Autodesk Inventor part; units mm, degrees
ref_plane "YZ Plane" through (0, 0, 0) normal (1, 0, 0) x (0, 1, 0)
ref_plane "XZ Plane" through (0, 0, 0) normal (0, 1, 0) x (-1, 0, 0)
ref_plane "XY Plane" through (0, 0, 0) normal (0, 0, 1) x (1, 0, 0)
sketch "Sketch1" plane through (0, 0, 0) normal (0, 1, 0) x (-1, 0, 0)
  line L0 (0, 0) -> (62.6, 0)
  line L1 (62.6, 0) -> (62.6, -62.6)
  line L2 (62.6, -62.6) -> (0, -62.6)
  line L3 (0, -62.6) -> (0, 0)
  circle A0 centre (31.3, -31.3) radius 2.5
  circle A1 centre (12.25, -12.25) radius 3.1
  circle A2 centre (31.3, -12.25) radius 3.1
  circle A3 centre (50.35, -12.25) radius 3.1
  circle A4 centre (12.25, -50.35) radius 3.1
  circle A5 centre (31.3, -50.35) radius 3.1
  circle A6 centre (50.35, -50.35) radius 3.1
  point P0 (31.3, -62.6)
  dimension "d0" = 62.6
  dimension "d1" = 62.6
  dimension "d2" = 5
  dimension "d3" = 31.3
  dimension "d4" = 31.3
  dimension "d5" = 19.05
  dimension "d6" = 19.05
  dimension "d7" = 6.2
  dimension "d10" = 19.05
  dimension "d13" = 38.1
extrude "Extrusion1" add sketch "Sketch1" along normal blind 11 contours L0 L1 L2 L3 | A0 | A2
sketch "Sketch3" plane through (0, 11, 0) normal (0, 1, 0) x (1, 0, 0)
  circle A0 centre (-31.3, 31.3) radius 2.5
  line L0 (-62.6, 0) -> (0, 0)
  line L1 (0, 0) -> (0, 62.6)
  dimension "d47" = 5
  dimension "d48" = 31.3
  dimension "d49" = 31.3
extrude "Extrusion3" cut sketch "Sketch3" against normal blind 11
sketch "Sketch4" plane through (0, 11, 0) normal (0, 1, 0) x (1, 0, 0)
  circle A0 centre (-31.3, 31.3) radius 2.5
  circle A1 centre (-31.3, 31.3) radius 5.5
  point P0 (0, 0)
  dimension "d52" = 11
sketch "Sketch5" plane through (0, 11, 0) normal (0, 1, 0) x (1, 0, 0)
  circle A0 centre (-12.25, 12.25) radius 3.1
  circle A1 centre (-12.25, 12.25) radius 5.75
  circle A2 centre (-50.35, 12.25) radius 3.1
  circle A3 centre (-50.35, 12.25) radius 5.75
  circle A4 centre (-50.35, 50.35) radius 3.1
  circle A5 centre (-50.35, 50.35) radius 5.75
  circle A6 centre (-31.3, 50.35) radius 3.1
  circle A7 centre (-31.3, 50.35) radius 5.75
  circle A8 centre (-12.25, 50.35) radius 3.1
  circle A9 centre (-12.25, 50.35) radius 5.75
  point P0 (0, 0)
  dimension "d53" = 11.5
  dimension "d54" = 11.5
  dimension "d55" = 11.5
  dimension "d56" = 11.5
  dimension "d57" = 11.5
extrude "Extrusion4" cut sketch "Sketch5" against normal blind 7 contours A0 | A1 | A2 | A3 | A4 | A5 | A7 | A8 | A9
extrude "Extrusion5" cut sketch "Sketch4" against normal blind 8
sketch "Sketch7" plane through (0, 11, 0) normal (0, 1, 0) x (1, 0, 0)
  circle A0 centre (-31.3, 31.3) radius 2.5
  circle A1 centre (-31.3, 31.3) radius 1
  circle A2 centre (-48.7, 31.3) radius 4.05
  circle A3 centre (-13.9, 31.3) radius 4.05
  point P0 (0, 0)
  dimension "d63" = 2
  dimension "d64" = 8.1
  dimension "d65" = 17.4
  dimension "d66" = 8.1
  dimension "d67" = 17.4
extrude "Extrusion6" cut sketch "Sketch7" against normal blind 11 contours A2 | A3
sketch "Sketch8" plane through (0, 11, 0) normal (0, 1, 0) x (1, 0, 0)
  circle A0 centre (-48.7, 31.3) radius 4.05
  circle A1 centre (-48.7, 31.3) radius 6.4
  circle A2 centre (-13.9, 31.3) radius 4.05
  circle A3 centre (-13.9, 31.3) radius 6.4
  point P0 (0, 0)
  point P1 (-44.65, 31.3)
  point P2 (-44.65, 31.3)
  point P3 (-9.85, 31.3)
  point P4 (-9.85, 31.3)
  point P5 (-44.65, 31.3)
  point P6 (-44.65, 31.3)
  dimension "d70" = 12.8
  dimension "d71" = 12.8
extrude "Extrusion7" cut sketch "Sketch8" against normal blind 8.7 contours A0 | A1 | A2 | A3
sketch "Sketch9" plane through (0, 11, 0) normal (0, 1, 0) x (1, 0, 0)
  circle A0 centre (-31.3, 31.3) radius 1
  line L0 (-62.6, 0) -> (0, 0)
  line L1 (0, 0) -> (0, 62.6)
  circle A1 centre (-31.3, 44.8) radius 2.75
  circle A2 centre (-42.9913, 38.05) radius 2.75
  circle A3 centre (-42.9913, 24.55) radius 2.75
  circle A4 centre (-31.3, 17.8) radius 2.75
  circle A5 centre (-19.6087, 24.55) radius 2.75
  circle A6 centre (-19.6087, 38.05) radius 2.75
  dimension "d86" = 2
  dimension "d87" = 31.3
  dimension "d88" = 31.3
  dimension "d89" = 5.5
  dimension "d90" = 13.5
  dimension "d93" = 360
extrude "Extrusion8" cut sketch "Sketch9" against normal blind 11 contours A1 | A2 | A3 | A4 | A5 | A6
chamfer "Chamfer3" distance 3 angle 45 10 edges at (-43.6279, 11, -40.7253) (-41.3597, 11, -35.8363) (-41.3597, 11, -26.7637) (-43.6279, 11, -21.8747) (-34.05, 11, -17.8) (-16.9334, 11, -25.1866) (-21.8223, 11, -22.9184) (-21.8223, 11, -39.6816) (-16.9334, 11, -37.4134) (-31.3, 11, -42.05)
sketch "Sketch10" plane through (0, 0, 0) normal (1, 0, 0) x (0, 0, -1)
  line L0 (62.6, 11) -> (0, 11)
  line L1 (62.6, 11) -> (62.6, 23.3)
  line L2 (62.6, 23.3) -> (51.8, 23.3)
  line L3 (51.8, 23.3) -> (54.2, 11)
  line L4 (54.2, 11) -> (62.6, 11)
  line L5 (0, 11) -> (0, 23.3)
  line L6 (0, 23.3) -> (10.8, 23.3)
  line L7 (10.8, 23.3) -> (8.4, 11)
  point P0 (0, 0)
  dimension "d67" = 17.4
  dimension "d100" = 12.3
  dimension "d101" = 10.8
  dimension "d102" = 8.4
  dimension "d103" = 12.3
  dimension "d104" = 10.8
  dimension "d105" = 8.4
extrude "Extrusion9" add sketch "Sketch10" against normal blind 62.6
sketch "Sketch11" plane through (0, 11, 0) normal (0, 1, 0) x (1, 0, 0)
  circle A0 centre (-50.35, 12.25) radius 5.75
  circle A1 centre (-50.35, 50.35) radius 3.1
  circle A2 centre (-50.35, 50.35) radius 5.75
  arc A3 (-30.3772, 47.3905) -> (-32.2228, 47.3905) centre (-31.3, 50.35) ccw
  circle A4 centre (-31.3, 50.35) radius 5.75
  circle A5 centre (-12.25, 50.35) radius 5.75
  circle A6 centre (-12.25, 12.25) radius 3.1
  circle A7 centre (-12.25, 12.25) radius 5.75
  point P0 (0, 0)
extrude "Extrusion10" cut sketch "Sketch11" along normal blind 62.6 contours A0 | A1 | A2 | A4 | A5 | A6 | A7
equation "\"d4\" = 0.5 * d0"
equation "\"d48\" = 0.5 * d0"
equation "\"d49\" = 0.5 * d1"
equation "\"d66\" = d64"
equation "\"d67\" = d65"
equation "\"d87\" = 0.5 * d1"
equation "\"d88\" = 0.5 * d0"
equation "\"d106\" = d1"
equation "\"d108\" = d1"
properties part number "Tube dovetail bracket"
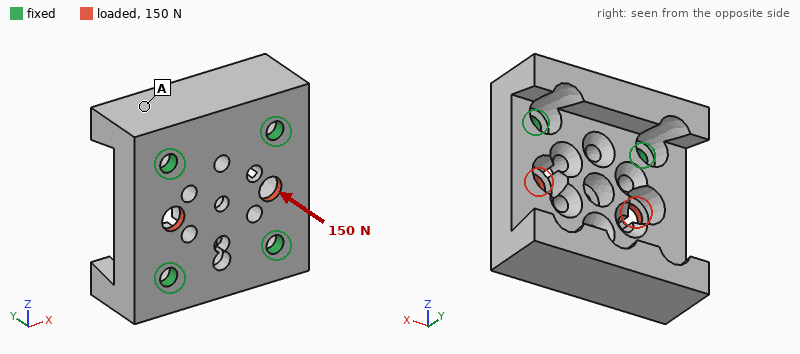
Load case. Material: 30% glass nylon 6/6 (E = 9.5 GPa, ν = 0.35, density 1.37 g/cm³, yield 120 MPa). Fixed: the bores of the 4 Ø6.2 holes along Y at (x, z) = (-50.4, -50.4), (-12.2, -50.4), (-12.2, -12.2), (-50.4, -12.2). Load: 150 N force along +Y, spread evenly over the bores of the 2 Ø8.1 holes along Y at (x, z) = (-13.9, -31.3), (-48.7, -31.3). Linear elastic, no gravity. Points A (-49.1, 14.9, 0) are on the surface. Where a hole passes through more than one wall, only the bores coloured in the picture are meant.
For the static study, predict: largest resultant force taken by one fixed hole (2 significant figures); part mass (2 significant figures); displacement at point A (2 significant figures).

44 N
64 g
2.4 µm
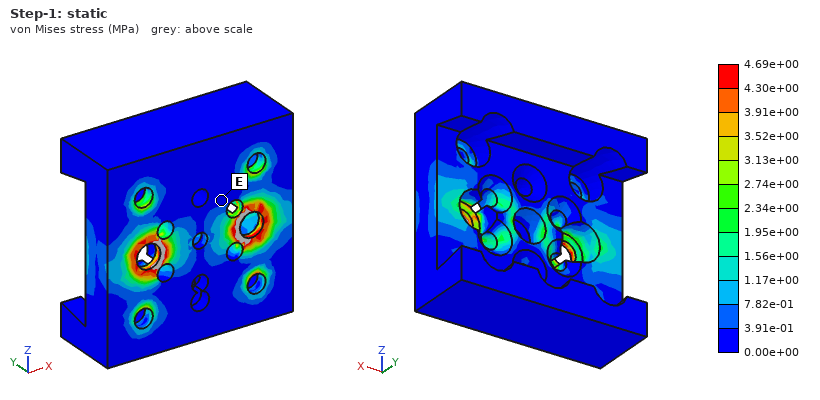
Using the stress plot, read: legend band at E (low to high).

0.00e+00 to 3.91e-01 MPa
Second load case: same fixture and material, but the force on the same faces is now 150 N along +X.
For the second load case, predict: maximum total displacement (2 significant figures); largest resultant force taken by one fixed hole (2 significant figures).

2.3 µm
38 N
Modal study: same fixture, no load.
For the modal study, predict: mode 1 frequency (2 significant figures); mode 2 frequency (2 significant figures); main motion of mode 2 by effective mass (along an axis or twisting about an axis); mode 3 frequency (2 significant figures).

4600 Hz
4900 Hz
along Z
6500 Hz
